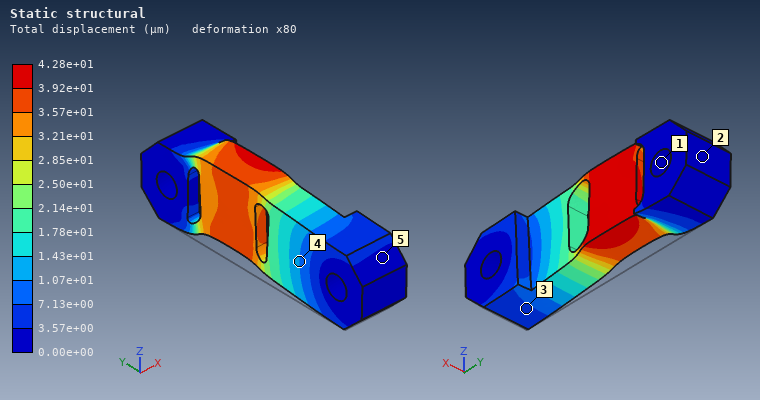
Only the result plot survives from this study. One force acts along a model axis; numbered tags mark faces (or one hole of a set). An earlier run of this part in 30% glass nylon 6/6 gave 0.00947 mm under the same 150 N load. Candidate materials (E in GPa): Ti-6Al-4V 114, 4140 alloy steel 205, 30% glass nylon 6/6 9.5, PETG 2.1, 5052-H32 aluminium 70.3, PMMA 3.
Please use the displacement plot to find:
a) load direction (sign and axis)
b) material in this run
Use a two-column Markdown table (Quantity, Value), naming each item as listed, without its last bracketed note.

| Quantity | Value |
|---|---|
| load direction | +Z |
| material in this run | PETG |
